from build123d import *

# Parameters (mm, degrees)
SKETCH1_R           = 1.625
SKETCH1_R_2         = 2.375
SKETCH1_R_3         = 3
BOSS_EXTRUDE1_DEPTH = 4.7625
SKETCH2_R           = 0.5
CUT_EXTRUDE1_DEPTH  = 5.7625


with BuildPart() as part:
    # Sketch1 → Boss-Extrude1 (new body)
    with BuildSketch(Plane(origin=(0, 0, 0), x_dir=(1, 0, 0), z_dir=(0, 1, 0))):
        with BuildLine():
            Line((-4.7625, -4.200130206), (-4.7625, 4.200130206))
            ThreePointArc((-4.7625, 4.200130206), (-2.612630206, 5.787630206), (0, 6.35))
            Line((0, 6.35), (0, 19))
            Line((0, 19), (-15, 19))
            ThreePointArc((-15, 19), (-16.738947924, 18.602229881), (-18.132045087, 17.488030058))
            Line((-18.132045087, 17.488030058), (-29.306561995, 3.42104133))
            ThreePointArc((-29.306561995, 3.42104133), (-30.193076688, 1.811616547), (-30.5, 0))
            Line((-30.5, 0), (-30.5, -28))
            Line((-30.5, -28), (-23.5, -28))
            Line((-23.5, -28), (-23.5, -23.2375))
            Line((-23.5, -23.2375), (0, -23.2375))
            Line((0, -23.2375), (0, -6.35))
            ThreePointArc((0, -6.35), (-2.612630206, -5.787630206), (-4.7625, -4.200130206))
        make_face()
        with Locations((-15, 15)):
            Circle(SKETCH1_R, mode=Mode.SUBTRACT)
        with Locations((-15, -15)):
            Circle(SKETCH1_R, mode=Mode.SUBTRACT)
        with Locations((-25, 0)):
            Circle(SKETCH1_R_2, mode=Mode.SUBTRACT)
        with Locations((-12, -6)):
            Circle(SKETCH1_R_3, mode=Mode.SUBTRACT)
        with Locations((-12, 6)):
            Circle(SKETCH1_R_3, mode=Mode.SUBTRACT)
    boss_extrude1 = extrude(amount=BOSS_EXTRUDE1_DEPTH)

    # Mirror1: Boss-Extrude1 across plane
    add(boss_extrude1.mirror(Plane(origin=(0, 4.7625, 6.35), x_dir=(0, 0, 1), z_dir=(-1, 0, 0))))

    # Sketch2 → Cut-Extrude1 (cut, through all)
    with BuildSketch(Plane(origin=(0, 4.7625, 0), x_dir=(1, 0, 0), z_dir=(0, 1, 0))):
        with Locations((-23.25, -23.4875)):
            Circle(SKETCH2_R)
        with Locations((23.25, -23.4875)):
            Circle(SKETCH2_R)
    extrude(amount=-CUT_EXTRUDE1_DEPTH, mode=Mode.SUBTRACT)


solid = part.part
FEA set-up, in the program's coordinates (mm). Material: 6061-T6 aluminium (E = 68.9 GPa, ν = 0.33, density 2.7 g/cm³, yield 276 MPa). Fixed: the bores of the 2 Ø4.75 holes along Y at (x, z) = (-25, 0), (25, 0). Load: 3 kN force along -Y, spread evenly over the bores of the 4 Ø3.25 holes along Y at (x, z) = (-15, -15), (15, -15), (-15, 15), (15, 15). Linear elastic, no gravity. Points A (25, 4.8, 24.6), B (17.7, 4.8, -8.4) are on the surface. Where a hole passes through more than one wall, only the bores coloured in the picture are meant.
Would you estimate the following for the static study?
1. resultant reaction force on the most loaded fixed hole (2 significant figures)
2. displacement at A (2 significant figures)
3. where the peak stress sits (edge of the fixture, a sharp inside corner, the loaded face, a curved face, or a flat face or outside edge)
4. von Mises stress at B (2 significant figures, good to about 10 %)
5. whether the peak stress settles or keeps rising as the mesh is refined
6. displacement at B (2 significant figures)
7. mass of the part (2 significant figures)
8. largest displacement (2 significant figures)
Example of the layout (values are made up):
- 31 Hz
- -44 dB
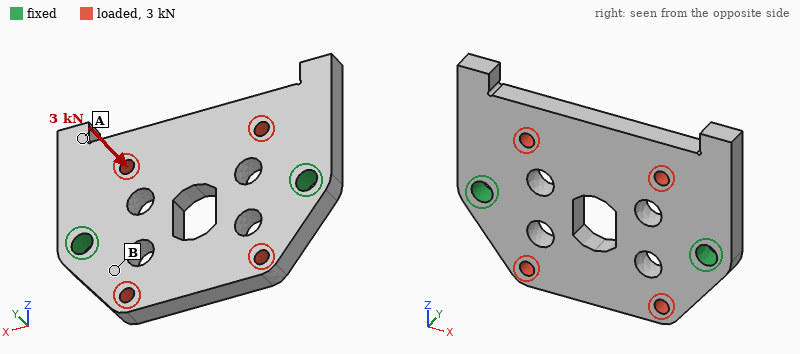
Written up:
- 1.5 kN
- 0.093 mm
- edge of the fixture
- 84 MPa
- keeps rising
- 0.048 mm
- 27 g
- 0.15 mm
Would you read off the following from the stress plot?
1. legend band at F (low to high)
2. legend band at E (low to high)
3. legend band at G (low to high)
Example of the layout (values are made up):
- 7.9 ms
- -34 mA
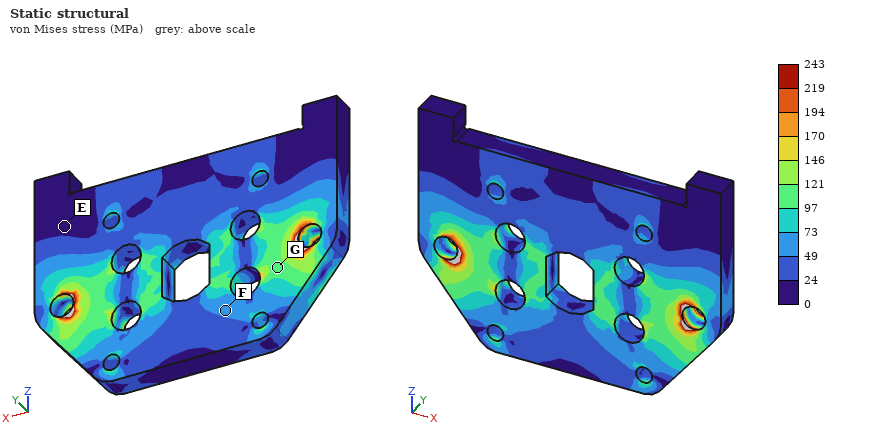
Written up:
- 49 to 73 MPa
- 0 to 24 MPa
- 97 to 121 MPa
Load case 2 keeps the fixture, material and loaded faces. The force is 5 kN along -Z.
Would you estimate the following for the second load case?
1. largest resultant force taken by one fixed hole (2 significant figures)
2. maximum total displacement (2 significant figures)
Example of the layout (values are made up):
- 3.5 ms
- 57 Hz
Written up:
- 2.5 kN
- 13 µm
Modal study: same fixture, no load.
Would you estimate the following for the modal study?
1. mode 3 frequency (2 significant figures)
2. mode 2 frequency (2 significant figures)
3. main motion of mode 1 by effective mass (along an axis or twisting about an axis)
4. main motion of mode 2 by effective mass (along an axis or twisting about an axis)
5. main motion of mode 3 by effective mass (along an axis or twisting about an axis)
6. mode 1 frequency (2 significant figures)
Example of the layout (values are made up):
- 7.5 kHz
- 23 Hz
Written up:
- 7500 Hz
- 6800 Hz
- along Y
- along Y
- twisting about Z
- 4700 Hz
